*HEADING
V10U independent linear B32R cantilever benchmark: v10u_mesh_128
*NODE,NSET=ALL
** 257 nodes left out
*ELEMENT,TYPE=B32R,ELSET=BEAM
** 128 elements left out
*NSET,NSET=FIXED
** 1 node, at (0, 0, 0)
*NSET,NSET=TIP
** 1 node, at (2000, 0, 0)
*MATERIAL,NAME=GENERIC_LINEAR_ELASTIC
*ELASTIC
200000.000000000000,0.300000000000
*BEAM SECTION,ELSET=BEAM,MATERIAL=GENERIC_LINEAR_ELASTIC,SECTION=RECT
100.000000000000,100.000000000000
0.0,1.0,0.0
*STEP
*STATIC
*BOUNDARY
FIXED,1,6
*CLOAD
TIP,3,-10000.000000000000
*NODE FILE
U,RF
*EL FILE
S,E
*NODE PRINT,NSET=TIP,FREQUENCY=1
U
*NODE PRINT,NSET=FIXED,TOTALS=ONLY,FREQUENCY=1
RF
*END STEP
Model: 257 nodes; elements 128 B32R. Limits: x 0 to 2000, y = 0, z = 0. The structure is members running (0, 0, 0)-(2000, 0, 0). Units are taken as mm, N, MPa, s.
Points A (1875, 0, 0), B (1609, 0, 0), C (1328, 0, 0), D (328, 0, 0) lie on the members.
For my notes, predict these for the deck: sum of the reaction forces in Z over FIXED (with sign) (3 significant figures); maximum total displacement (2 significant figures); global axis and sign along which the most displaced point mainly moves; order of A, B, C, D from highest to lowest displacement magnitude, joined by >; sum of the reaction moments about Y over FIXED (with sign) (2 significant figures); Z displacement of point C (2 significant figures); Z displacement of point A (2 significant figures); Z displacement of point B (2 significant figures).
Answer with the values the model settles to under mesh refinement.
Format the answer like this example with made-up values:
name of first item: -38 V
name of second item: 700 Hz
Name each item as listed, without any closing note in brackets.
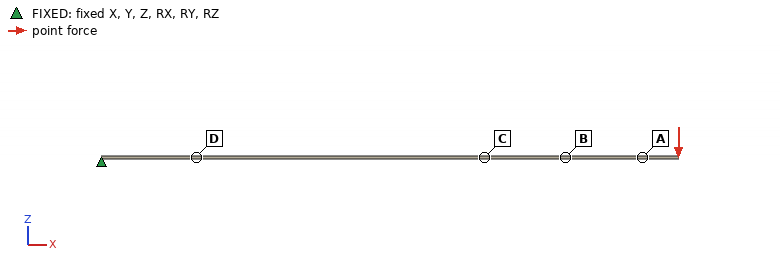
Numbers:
sum of the reaction forces in Z over FIXED (with sign): 10000 N
maximum total displacement: 16 mm
global axis and sign along which the most displaced point mainly moves: -Z
order of A, B, C, D from highest to lowest displacement magnitude, joined by >: A > B > C > D
sum of the reaction moments about Y over FIXED (with sign): -2.0e+07 N·mm
Z displacement of point C: -8.3 mm
Z displacement of point A: -15 mm
Z displacement of point B: -11 mm
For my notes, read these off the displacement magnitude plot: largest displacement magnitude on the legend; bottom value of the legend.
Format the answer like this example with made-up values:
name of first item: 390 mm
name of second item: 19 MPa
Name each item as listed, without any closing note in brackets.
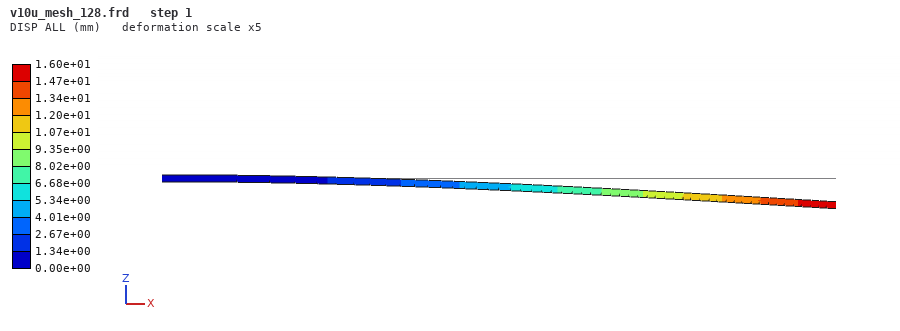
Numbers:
largest displacement magnitude on the legend: 1.60e+01 mm
bottom value of the legend: 0.00e+00 mm
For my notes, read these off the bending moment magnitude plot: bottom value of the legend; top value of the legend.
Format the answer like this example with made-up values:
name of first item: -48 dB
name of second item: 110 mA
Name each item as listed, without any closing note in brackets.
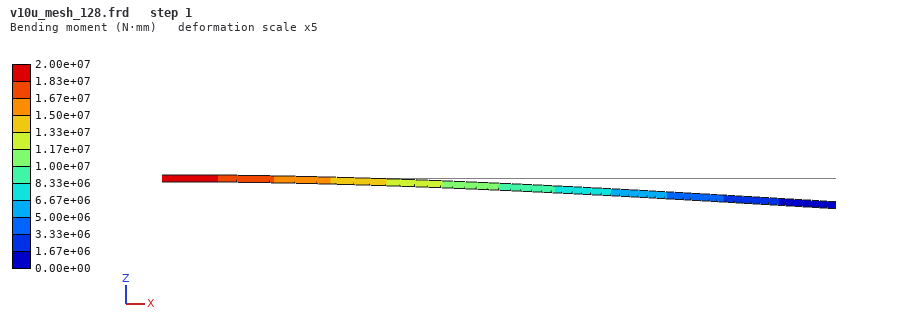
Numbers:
bottom value of the legend: 0.00e+00 N·mm
top value of the legend: 2.00e+07 N·mm
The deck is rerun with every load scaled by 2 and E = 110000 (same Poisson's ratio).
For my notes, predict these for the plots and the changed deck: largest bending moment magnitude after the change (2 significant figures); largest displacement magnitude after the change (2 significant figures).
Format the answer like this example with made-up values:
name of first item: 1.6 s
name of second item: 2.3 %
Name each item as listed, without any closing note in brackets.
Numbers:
largest bending moment magnitude after the change: 4.0e+07 N·mm
largest displacement magnitude after the change: 58 mm
